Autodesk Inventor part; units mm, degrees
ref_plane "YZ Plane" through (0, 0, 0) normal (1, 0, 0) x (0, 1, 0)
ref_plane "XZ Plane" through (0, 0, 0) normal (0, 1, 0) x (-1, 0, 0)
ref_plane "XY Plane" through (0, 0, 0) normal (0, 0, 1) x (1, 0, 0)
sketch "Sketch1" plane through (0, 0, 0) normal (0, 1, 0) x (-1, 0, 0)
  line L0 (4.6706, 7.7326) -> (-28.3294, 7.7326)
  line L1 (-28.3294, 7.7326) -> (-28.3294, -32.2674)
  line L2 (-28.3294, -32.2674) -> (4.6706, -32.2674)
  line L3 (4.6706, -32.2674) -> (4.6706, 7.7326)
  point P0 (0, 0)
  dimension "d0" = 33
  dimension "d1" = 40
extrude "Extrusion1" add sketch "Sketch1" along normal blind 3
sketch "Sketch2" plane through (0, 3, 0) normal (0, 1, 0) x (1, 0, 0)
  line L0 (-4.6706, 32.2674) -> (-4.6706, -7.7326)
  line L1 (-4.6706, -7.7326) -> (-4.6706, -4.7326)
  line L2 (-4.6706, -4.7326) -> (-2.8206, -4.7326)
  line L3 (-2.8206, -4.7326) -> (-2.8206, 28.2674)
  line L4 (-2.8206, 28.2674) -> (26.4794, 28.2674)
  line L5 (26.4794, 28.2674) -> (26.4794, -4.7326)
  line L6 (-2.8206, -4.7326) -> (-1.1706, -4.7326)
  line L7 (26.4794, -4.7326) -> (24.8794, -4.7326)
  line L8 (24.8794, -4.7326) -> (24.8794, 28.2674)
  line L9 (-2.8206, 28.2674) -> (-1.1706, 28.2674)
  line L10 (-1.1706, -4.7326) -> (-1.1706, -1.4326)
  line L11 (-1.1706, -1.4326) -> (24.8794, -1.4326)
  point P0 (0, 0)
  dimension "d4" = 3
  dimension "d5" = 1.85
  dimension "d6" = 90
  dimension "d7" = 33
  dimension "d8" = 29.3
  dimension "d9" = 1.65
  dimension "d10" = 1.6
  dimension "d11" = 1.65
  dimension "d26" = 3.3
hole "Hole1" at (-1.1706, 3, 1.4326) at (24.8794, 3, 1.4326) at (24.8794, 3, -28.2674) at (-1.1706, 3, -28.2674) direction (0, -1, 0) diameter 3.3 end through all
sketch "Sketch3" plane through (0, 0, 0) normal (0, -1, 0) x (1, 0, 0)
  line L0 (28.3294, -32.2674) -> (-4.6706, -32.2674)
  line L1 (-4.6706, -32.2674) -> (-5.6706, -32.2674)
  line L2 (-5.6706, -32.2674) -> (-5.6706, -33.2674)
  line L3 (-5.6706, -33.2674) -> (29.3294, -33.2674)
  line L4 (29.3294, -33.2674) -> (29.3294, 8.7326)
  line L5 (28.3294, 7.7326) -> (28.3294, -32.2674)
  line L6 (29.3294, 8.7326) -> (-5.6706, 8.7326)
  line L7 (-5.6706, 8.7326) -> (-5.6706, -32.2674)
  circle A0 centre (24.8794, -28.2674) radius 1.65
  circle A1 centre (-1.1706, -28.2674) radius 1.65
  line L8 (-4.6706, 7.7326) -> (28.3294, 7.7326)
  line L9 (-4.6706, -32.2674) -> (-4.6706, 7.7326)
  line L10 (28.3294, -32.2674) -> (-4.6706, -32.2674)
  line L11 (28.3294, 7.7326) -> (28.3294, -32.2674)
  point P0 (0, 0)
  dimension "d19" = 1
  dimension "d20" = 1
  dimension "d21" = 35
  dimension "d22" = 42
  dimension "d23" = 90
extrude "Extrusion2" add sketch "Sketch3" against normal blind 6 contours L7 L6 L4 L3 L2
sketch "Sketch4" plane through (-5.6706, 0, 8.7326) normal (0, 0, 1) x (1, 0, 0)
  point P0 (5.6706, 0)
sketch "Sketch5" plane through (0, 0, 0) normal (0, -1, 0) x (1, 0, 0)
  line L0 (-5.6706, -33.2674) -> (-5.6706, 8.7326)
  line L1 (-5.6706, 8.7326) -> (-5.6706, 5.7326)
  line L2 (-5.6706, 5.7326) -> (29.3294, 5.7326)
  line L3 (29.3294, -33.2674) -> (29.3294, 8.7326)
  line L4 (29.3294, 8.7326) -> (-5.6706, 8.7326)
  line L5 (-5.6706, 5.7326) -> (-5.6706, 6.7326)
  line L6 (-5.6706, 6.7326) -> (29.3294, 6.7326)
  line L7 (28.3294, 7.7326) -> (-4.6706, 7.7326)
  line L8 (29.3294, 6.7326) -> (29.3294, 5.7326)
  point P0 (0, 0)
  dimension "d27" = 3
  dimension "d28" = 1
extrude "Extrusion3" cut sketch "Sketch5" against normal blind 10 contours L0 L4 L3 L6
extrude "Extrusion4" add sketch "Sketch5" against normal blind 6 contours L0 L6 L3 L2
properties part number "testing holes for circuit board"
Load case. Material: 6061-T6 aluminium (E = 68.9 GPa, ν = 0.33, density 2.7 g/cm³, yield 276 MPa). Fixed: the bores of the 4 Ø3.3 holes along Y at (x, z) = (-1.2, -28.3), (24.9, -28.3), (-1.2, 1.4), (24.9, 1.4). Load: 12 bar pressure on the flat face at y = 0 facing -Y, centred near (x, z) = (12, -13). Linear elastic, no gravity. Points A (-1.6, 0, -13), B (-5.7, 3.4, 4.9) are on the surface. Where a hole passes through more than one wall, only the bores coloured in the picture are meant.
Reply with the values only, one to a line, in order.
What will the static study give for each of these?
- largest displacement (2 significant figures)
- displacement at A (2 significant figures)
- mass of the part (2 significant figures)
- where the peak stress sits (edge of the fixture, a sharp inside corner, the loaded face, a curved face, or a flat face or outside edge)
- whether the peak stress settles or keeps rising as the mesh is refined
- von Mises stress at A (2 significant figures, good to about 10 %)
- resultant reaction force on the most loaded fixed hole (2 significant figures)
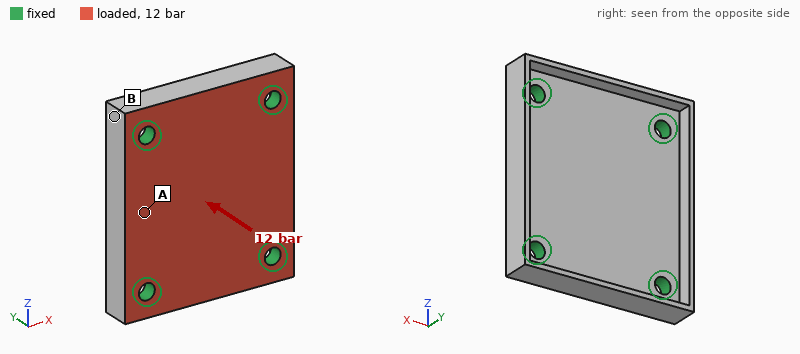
26 µm
14 µm
12 g
edge of the fixture
keeps rising
22 MPa
410 N
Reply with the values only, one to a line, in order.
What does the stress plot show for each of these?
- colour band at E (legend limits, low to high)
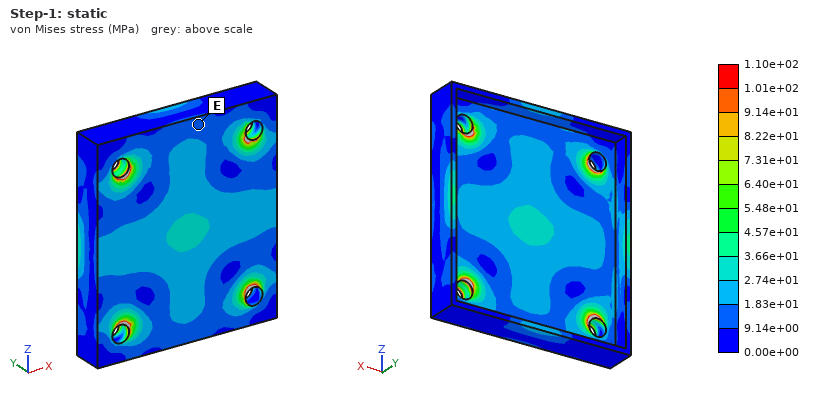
9.14e+00 to 1.83e+01 MPa
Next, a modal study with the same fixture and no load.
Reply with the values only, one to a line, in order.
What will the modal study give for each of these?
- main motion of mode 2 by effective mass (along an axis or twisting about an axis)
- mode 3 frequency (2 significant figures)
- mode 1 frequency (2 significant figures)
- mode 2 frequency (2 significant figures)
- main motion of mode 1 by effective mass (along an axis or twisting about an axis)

twisting about Z
24 kHz
15 kHz
22 kHz
along Y
